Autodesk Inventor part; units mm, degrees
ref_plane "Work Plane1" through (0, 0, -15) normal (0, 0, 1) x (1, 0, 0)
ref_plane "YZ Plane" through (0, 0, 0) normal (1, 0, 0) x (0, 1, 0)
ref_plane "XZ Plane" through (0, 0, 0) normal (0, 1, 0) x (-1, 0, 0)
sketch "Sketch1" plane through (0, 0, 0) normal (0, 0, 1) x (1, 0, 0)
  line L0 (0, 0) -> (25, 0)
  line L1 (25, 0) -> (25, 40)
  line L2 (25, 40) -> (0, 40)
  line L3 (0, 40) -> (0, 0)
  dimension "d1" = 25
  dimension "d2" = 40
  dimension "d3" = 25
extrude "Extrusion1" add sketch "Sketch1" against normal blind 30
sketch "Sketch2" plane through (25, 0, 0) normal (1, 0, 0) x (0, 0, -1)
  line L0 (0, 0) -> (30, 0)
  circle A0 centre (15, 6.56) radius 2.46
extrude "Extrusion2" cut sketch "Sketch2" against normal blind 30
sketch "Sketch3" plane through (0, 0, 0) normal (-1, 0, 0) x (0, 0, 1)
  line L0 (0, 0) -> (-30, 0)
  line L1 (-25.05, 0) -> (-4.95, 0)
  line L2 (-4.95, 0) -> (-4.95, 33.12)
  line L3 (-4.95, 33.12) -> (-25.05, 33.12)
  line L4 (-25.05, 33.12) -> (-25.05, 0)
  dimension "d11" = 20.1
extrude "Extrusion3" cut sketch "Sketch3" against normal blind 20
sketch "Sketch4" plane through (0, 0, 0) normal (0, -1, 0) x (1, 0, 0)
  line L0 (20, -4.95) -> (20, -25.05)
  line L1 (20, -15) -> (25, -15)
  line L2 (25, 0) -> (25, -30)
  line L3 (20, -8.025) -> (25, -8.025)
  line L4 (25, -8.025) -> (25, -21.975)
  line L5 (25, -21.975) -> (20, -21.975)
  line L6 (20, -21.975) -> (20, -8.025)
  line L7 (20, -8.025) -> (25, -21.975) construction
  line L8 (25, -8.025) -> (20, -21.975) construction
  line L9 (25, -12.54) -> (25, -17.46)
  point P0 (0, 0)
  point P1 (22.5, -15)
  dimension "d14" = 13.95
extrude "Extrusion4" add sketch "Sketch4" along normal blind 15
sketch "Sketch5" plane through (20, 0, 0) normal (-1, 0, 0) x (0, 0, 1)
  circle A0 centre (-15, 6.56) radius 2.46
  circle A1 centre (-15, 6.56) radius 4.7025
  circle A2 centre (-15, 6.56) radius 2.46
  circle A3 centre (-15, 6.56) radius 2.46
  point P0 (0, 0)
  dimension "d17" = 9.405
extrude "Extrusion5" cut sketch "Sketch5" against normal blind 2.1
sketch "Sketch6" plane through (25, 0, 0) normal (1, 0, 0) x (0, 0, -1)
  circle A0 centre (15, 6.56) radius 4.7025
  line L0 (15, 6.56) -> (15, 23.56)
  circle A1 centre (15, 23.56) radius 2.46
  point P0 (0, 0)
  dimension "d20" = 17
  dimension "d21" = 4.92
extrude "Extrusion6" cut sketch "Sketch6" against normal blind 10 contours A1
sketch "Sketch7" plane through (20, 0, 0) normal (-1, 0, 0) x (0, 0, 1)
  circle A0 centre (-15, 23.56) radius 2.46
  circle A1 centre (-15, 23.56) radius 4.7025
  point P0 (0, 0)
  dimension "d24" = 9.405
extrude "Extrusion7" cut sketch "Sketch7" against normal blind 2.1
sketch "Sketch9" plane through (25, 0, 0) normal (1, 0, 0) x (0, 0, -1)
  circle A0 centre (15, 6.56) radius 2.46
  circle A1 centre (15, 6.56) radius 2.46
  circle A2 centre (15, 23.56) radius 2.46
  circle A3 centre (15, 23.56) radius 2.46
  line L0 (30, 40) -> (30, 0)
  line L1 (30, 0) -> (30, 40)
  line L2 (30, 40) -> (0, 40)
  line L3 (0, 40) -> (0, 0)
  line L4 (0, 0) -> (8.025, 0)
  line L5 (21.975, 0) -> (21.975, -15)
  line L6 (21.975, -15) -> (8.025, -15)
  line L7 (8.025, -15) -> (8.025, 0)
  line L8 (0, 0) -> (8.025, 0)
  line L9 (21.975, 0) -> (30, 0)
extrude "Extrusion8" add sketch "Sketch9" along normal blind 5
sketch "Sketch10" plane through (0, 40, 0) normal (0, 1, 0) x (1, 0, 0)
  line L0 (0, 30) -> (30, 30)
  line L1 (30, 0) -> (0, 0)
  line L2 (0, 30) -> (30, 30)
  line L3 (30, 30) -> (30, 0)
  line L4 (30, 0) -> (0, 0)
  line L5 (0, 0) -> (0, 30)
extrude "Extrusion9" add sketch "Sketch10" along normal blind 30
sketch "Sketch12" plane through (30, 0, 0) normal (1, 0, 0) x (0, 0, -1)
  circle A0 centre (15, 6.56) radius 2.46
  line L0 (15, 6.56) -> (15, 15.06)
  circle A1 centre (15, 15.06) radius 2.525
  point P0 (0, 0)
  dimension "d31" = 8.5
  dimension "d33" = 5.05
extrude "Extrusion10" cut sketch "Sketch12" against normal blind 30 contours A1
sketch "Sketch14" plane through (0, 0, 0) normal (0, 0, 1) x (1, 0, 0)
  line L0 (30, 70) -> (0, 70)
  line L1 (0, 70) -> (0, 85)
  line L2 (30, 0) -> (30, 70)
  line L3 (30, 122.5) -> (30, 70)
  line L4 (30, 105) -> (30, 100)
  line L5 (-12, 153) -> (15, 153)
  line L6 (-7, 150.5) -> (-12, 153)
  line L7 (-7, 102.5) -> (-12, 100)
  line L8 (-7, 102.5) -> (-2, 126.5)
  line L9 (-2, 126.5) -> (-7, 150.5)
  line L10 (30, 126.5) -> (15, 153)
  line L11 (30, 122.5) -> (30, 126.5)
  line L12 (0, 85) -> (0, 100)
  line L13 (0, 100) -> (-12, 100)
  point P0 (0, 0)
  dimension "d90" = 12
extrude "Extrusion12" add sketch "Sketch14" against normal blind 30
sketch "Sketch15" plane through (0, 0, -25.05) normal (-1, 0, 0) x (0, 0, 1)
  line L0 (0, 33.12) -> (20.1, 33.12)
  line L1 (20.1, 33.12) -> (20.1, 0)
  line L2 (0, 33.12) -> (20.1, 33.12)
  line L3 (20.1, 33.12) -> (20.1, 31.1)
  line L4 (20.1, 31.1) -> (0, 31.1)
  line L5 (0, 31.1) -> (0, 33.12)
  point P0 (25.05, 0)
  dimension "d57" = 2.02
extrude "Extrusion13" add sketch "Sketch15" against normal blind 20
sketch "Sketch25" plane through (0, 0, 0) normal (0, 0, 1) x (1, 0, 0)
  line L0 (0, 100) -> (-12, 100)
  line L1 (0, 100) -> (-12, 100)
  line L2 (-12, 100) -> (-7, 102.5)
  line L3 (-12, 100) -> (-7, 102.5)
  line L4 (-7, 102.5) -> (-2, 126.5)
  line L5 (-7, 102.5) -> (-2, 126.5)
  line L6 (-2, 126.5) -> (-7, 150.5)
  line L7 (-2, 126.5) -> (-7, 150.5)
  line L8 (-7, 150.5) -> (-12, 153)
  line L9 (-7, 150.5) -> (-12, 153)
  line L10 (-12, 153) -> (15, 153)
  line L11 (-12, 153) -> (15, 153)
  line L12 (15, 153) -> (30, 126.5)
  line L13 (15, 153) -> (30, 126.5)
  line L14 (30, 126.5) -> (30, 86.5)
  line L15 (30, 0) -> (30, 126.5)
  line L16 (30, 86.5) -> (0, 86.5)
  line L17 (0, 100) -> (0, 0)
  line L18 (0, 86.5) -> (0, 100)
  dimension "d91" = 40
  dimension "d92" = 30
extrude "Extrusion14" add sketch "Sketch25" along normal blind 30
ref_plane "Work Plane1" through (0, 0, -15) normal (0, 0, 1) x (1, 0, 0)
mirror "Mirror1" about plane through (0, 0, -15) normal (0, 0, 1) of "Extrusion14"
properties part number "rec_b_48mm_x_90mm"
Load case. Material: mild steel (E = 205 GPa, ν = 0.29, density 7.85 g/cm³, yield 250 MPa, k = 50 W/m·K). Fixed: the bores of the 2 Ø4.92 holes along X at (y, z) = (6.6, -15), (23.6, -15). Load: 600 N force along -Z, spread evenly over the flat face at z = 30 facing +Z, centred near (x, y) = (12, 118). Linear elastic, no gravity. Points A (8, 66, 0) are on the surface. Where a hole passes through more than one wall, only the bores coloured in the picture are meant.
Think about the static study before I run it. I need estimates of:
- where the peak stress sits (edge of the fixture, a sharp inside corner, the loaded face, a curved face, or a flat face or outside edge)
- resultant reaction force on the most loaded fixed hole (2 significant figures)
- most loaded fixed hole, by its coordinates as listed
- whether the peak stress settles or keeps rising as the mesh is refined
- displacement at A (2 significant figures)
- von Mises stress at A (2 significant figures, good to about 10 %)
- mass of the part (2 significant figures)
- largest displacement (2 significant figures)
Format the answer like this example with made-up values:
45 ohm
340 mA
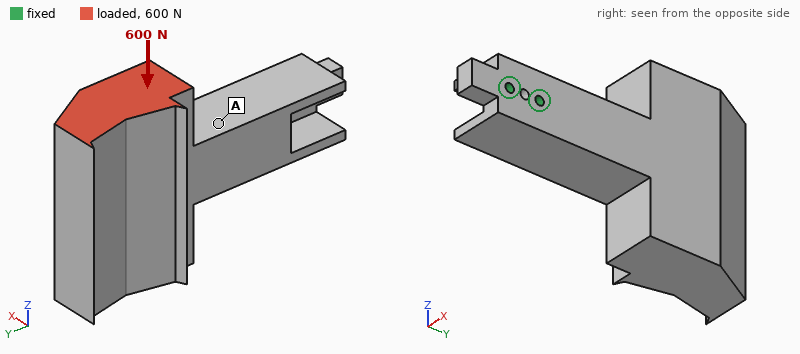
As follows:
edge of the fixture
3.0 kN
(23.6, -15)
keeps rising
16 µm
6.9 MPa
2.0 kg
57 µm
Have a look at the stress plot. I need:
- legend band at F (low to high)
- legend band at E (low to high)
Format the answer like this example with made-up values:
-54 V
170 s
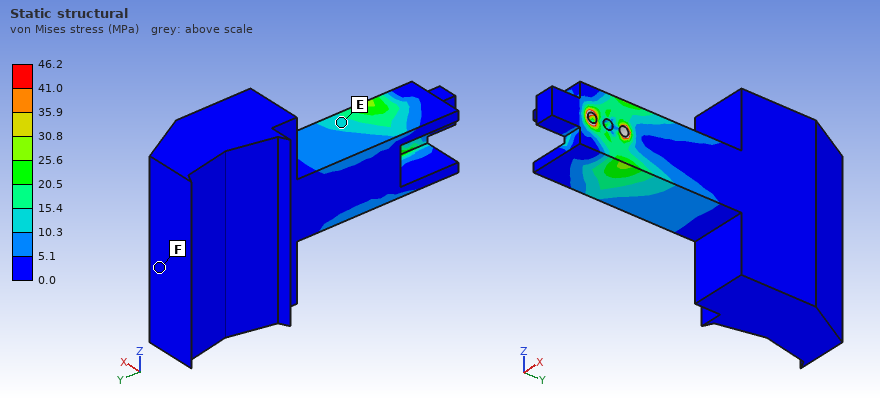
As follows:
0.0 to 5.1 MPa
10.3 to 15.4 MPa
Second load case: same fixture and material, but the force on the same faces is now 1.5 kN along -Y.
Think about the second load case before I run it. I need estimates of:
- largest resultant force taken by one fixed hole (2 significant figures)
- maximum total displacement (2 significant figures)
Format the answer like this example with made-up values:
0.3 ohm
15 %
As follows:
3.2 kN
86 µm
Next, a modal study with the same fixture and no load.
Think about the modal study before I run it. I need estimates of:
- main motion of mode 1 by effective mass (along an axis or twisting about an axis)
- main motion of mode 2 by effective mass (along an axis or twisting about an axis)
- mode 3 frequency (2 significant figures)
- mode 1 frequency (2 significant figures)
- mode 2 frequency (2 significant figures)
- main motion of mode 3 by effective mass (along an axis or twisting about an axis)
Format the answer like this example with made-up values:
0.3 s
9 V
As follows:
along X
along Z
980 Hz
430 Hz
490 Hz
twisting about Y
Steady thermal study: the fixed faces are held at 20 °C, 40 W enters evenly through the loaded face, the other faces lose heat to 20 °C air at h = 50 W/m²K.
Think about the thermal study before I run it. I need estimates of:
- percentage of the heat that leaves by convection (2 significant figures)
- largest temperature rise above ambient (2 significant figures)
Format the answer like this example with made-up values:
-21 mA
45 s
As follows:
79 %
38 K
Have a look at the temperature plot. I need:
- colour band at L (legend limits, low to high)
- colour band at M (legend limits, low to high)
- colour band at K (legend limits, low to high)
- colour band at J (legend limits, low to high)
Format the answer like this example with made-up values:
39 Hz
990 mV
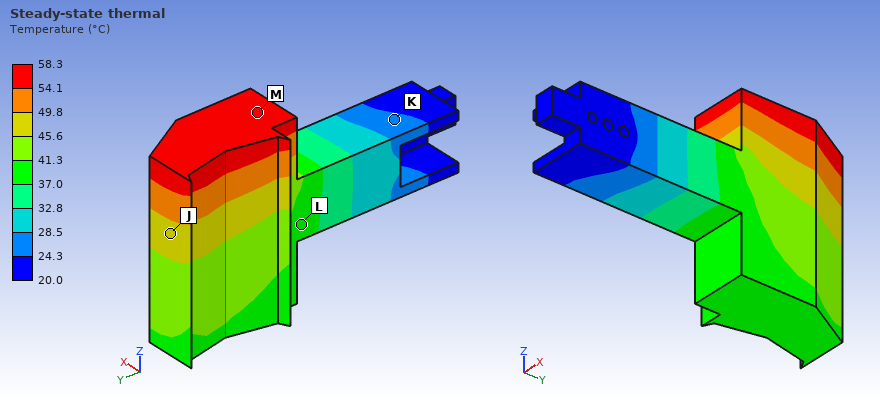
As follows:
37.0 to 41.3 °C
54.1 to 58.3 °C
24.3 to 28.5 °C
45.6 to 49.8 °C
